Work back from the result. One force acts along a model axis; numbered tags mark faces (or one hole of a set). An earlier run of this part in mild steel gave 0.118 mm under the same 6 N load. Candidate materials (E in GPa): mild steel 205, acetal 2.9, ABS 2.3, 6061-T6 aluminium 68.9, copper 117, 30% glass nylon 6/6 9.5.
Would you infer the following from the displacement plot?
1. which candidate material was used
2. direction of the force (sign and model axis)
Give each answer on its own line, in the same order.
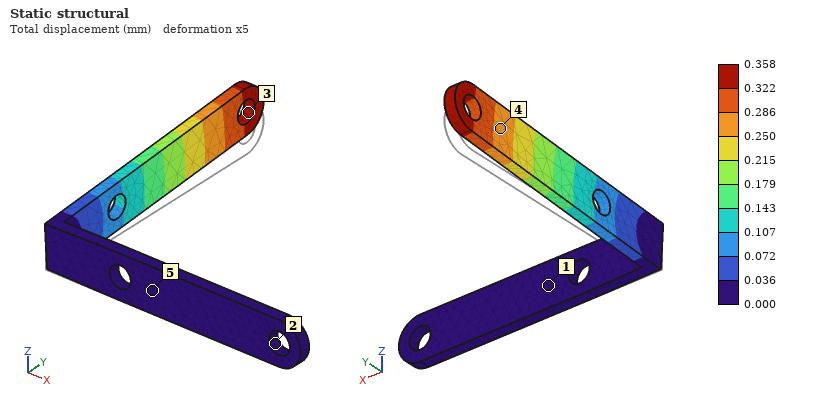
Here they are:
6061-T6 aluminium
+Z
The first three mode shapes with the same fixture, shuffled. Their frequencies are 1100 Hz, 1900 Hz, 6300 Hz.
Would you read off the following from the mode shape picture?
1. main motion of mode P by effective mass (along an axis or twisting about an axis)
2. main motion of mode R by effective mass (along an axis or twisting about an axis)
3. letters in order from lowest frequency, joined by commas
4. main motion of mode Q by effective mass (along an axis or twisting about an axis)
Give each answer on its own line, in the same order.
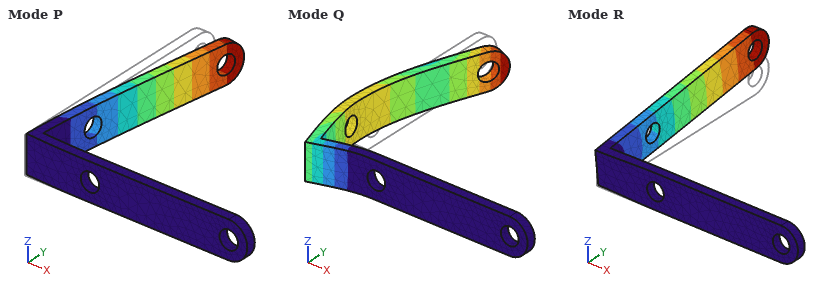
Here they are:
along X
along Z
P, R, Q
along Y
